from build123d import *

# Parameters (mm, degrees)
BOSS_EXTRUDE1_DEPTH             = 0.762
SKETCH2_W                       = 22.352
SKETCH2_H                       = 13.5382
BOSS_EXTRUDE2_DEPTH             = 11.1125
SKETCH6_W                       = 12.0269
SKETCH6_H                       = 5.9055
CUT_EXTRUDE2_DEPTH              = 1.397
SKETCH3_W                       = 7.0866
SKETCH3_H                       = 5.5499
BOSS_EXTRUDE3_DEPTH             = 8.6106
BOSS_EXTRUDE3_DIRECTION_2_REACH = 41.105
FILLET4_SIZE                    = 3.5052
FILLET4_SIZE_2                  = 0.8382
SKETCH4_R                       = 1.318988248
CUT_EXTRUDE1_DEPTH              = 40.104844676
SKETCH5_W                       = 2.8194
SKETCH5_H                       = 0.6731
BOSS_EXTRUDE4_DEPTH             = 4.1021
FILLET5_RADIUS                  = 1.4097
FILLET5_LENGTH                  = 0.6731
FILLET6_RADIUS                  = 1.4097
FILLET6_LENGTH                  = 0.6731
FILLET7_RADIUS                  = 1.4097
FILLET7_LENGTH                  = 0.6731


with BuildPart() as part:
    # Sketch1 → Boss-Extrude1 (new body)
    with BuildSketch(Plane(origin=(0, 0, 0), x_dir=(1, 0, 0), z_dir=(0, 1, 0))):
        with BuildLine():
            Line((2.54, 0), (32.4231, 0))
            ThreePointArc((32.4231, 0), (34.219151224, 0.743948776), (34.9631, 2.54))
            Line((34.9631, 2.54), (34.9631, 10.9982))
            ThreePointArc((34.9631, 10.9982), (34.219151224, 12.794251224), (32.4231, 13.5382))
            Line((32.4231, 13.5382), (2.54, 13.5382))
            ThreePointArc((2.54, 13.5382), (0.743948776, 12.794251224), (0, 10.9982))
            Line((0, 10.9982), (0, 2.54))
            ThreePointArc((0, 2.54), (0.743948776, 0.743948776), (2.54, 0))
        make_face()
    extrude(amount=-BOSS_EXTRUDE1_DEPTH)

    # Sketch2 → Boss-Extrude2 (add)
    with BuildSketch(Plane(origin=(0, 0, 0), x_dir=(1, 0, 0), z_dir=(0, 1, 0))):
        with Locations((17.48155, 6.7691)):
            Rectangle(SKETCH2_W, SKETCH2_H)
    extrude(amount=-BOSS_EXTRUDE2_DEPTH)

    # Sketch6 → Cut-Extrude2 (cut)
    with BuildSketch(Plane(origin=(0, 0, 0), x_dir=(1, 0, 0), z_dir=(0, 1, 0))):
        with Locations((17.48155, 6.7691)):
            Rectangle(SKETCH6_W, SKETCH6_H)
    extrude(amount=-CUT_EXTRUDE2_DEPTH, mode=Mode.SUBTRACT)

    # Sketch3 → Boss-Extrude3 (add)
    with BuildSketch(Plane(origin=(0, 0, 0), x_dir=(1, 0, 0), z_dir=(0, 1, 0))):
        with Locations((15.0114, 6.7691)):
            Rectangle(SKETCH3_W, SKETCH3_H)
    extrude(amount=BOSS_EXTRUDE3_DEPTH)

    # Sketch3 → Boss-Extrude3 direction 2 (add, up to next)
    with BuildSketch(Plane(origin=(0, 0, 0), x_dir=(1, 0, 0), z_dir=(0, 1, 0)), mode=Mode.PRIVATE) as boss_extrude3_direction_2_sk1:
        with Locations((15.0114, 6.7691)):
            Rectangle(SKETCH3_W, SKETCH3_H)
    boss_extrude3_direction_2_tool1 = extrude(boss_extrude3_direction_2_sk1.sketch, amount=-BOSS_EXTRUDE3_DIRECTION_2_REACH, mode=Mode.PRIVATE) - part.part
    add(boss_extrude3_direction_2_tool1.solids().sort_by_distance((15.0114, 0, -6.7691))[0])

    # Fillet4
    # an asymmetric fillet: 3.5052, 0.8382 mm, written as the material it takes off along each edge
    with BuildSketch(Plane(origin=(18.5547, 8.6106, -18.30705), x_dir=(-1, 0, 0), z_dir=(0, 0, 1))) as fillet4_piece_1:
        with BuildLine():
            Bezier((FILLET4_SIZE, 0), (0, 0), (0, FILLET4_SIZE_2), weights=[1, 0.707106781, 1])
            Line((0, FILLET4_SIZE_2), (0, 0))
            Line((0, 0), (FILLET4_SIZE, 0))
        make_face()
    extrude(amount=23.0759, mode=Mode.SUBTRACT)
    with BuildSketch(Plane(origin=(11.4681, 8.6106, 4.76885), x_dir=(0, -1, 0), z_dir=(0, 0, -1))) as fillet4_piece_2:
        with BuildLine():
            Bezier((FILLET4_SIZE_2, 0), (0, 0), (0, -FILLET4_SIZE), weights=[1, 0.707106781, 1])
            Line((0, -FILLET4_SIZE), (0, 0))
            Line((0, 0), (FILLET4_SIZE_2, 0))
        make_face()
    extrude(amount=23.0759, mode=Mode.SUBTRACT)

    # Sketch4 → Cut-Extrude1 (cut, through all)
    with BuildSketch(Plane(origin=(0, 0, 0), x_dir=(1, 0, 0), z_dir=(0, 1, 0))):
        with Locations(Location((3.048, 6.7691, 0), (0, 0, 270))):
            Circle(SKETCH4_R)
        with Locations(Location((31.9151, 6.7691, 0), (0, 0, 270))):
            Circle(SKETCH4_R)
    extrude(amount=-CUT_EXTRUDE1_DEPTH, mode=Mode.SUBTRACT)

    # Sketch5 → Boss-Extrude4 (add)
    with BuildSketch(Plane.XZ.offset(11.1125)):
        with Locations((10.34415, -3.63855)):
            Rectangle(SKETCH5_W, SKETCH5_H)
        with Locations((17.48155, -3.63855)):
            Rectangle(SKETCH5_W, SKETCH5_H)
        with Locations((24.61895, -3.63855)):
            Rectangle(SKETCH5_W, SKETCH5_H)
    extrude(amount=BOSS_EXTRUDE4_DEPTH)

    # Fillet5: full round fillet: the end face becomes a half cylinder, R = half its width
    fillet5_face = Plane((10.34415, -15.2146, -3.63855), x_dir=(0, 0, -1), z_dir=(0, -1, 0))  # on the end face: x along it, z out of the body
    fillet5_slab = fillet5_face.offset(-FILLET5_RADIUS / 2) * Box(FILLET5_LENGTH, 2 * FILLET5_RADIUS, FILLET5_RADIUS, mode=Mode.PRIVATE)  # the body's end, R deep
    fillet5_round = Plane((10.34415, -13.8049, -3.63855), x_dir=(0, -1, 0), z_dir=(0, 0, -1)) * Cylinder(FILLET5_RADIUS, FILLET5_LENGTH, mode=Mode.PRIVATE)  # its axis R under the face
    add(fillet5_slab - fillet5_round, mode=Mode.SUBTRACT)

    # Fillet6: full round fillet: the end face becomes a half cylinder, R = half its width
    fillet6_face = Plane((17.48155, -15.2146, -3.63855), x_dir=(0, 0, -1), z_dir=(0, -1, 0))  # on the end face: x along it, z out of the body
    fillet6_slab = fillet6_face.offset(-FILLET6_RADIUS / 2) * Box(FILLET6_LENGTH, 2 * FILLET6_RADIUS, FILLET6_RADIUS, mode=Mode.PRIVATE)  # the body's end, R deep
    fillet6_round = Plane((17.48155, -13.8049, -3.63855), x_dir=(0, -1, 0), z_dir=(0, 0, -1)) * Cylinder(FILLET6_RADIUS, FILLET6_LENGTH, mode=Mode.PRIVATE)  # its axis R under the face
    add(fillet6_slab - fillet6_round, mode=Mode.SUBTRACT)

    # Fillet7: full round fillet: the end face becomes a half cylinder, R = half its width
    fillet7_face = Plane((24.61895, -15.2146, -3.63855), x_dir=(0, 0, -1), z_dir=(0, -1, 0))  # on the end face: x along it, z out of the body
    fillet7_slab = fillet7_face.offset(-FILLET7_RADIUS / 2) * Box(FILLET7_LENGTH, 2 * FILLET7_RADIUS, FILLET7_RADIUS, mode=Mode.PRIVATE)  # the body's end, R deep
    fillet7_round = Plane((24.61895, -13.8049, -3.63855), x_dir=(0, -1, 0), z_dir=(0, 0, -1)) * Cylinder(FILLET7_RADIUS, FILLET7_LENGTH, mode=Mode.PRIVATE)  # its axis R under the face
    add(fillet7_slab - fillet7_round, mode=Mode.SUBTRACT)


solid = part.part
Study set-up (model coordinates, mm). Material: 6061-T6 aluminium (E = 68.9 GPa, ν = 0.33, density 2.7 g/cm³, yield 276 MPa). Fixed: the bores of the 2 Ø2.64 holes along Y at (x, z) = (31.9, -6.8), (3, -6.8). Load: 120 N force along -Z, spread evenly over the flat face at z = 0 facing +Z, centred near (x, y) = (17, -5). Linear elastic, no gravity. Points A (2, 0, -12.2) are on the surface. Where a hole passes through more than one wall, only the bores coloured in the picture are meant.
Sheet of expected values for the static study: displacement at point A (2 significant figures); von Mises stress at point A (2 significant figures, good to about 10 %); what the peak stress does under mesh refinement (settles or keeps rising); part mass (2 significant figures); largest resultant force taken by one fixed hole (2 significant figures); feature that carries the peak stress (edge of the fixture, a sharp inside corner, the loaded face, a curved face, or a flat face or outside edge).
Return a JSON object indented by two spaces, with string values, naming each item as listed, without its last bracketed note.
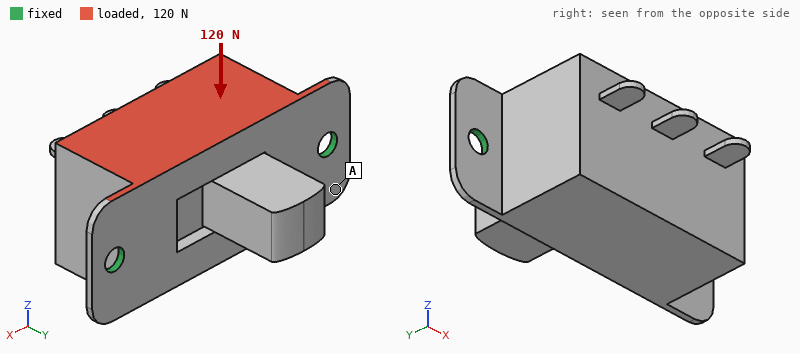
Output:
{
  "displacement at point A": "0.027 mm",
  "von Mises stress at point A": "27 MPa",
  "what the peak stress does under mesh refinement": "keeps rising",
  "part mass": "10 g",
  "largest resultant force taken by one fixed hole": "60 N",
  "feature that carries the peak stress": "edge of the fixture"
}
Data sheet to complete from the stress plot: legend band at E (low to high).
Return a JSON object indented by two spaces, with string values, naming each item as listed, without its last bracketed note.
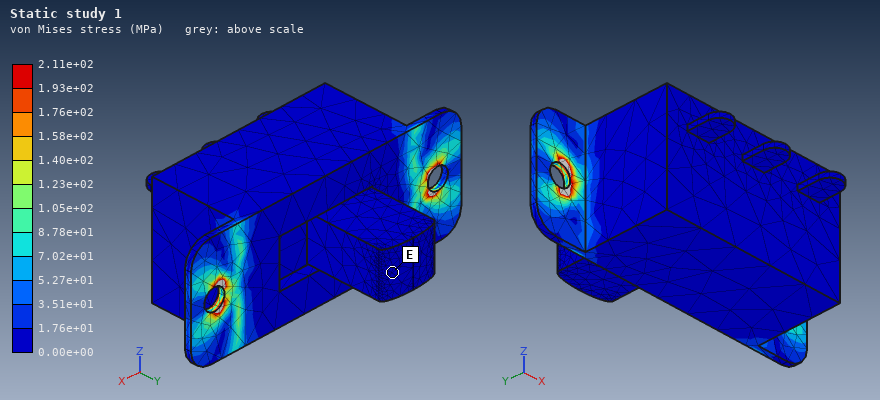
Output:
{
  "legend band at E": "0.00e+00 to 1.76e+01 MPa"
}
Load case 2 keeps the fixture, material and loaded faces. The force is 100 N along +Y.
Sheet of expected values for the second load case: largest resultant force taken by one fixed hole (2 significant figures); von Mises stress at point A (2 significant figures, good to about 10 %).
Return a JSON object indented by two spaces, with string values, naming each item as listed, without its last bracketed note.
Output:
{
  "largest resultant force taken by one fixed hole": "58 N",
  "von Mises stress at point A": "28 MPa"
}
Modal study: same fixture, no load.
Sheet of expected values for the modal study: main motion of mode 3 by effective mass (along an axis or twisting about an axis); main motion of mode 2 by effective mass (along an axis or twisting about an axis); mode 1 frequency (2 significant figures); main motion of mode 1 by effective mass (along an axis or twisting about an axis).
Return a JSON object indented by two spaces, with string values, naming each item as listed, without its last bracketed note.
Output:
{
  "main motion of mode 3 by effective mass": "along X",
  "main motion of mode 2 by effective mass": "along Y",
  "mode 1 frequency": "1800 Hz",
  "main motion of mode 1 by effective mass": "along Z"
}
